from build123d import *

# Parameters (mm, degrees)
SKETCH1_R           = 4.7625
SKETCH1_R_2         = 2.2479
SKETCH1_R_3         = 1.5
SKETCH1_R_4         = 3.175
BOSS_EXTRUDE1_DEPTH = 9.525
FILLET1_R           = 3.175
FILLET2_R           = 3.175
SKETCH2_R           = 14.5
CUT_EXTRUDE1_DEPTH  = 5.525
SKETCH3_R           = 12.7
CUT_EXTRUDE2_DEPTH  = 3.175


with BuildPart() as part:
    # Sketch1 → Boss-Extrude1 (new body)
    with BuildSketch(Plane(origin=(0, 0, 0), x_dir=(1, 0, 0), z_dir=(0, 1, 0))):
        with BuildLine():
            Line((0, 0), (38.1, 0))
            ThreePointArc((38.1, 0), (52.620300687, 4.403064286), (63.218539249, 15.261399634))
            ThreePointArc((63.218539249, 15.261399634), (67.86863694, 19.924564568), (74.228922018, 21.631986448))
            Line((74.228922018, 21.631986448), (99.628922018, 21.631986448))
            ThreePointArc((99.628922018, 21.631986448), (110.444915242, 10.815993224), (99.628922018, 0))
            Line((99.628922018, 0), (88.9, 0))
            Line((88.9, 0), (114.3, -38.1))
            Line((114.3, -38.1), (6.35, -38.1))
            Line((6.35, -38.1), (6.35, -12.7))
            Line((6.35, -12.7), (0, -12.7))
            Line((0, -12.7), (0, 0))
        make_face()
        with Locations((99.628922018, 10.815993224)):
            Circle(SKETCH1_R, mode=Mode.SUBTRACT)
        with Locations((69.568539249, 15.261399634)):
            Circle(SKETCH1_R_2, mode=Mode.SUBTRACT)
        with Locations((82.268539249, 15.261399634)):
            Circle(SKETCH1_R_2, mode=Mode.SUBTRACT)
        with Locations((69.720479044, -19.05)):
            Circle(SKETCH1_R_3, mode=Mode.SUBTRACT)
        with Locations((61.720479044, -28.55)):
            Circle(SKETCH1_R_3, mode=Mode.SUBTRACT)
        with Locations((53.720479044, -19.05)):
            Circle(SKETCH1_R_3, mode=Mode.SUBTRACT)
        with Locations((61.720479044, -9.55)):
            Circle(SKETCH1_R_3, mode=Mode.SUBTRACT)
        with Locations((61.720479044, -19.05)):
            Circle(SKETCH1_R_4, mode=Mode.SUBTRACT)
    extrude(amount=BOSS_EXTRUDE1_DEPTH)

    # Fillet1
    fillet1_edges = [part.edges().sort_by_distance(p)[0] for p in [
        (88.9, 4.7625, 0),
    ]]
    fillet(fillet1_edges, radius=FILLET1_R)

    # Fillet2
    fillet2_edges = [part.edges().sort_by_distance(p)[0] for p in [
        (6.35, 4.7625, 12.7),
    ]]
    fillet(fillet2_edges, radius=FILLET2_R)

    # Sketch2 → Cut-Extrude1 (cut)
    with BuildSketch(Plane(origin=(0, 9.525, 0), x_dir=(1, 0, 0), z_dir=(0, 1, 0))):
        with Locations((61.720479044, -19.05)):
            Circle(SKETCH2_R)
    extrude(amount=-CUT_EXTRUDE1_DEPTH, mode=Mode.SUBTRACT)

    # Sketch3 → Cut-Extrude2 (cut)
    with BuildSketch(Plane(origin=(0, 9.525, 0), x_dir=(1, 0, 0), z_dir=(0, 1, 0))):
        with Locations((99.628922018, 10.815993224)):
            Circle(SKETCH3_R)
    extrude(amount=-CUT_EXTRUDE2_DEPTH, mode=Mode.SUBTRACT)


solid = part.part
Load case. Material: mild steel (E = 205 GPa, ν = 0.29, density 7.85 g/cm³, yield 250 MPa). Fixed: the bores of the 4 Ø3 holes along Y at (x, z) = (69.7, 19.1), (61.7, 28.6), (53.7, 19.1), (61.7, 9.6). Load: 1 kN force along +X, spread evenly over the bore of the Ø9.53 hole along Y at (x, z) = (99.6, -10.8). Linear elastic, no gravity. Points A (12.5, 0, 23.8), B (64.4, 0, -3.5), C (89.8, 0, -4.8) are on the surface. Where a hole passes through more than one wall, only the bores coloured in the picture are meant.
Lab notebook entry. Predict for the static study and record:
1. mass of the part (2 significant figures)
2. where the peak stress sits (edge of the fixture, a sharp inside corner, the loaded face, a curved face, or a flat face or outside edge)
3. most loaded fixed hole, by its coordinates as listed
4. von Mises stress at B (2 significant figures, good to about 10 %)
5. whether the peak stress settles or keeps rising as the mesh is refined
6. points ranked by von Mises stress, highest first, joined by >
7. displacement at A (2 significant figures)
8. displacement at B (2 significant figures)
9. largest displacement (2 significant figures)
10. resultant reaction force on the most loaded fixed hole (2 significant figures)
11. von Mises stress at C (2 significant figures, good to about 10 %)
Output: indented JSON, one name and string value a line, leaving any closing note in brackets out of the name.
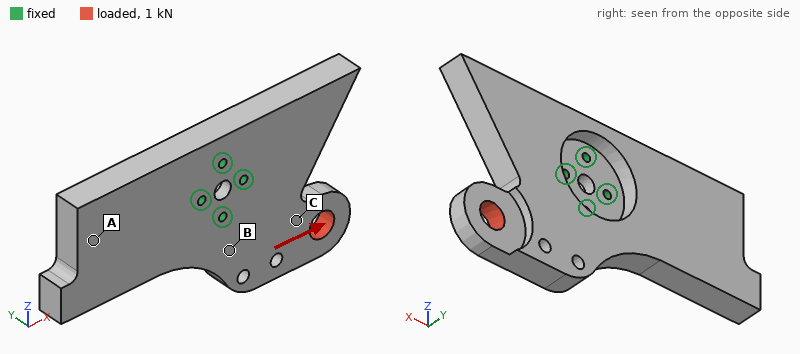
{
  "mass of the part": "310 g",
  "where the peak stress sits": "edge of the fixture",
  "most loaded fixed hole, by its coordinates as listed": "(61.7, 9.6)",
  "von Mises stress at B": "6.7 MPa",
  "whether the peak stress settles or keeps rising as the mesh is refined": "keeps rising",
  "points ranked by von Mises stress, highest first, joined by >": "C > B > A",
  "displacement at A": "4.3 µm",
  "displacement at B": "2.3 µm",
  "largest displacement": "7.9 µm",
  "resultant reaction force on the most loaded fixed hole": "1.2 kN",
  "von Mises stress at C": "10 MPa"
}
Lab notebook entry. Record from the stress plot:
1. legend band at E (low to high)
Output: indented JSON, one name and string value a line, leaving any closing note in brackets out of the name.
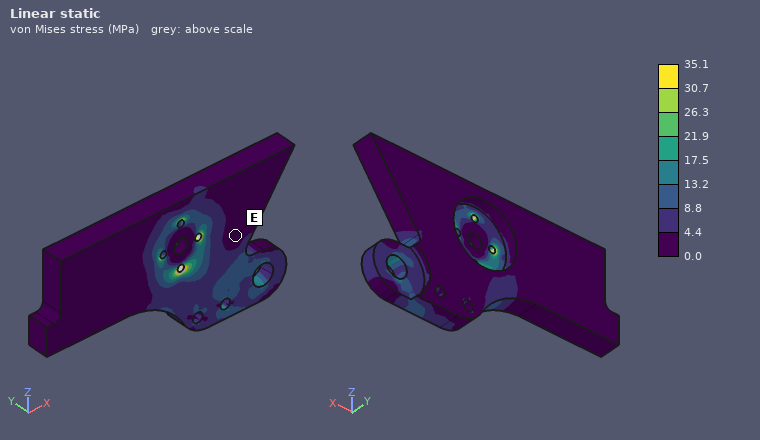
{
  "legend band at E": "0.0 to 4.4 MPa"
}
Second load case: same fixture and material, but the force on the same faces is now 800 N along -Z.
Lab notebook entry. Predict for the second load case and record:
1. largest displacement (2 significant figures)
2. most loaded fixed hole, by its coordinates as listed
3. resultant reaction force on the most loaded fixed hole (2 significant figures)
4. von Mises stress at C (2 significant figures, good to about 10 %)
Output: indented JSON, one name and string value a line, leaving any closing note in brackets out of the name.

{
  "largest displacement": "11 µm",
  "most loaded fixed hole, by its coordinates as listed": "(69.7, 19.1)",
  "resultant reaction force on the most loaded fixed hole": "1.1 kN",
  "von Mises stress at C": "11 MPa"
}
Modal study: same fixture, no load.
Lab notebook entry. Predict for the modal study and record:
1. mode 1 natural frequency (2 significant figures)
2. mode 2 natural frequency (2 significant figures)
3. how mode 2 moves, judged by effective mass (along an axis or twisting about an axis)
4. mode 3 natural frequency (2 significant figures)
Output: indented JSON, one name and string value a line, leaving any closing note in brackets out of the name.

{
  "mode 1 natural frequency": "1700 Hz",
  "mode 2 natural frequency": "2800 Hz",
  "how mode 2 moves, judged by effective mass": "along Y",
  "mode 3 natural frequency": "3500 Hz"
}
